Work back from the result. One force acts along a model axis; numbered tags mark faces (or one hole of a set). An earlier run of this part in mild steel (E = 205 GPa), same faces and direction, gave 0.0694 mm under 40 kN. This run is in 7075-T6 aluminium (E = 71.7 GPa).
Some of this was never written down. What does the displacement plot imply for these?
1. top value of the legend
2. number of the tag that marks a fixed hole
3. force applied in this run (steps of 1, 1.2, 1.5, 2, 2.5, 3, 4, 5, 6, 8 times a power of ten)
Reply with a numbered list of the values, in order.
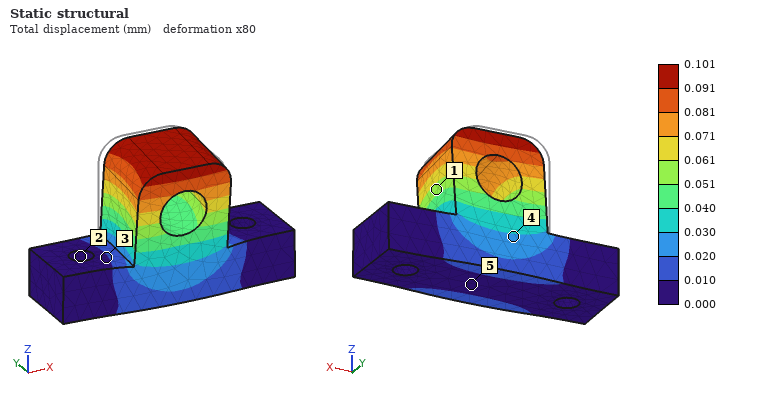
1. 0.101 mm
2. 2
3. 20 kN
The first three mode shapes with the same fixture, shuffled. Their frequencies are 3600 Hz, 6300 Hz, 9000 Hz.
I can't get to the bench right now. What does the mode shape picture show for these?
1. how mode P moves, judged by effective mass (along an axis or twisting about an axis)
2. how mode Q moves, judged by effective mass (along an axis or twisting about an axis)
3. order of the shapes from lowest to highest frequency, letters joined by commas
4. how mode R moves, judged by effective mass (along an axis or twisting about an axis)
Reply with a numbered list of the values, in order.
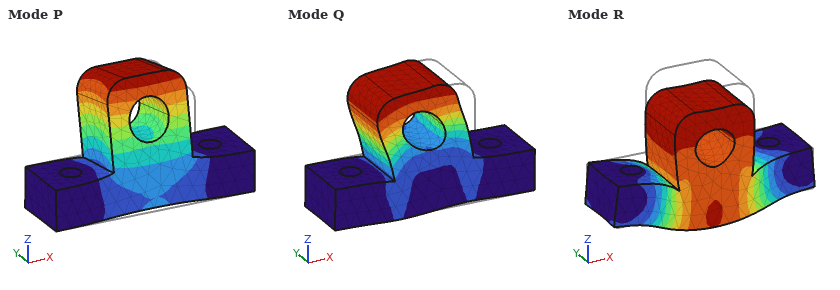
1. along Y
2. along X
3. P, Q, R
4. along Z
